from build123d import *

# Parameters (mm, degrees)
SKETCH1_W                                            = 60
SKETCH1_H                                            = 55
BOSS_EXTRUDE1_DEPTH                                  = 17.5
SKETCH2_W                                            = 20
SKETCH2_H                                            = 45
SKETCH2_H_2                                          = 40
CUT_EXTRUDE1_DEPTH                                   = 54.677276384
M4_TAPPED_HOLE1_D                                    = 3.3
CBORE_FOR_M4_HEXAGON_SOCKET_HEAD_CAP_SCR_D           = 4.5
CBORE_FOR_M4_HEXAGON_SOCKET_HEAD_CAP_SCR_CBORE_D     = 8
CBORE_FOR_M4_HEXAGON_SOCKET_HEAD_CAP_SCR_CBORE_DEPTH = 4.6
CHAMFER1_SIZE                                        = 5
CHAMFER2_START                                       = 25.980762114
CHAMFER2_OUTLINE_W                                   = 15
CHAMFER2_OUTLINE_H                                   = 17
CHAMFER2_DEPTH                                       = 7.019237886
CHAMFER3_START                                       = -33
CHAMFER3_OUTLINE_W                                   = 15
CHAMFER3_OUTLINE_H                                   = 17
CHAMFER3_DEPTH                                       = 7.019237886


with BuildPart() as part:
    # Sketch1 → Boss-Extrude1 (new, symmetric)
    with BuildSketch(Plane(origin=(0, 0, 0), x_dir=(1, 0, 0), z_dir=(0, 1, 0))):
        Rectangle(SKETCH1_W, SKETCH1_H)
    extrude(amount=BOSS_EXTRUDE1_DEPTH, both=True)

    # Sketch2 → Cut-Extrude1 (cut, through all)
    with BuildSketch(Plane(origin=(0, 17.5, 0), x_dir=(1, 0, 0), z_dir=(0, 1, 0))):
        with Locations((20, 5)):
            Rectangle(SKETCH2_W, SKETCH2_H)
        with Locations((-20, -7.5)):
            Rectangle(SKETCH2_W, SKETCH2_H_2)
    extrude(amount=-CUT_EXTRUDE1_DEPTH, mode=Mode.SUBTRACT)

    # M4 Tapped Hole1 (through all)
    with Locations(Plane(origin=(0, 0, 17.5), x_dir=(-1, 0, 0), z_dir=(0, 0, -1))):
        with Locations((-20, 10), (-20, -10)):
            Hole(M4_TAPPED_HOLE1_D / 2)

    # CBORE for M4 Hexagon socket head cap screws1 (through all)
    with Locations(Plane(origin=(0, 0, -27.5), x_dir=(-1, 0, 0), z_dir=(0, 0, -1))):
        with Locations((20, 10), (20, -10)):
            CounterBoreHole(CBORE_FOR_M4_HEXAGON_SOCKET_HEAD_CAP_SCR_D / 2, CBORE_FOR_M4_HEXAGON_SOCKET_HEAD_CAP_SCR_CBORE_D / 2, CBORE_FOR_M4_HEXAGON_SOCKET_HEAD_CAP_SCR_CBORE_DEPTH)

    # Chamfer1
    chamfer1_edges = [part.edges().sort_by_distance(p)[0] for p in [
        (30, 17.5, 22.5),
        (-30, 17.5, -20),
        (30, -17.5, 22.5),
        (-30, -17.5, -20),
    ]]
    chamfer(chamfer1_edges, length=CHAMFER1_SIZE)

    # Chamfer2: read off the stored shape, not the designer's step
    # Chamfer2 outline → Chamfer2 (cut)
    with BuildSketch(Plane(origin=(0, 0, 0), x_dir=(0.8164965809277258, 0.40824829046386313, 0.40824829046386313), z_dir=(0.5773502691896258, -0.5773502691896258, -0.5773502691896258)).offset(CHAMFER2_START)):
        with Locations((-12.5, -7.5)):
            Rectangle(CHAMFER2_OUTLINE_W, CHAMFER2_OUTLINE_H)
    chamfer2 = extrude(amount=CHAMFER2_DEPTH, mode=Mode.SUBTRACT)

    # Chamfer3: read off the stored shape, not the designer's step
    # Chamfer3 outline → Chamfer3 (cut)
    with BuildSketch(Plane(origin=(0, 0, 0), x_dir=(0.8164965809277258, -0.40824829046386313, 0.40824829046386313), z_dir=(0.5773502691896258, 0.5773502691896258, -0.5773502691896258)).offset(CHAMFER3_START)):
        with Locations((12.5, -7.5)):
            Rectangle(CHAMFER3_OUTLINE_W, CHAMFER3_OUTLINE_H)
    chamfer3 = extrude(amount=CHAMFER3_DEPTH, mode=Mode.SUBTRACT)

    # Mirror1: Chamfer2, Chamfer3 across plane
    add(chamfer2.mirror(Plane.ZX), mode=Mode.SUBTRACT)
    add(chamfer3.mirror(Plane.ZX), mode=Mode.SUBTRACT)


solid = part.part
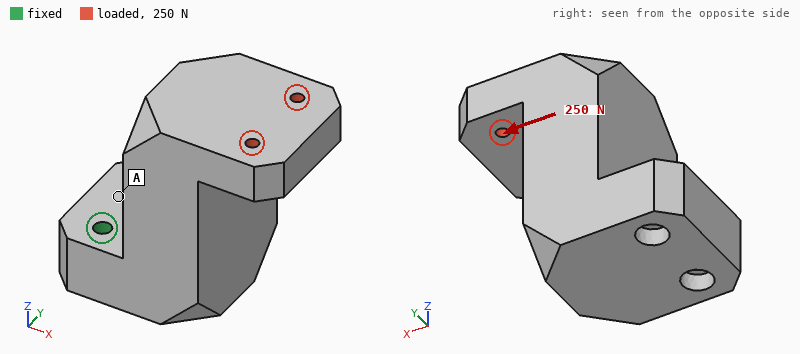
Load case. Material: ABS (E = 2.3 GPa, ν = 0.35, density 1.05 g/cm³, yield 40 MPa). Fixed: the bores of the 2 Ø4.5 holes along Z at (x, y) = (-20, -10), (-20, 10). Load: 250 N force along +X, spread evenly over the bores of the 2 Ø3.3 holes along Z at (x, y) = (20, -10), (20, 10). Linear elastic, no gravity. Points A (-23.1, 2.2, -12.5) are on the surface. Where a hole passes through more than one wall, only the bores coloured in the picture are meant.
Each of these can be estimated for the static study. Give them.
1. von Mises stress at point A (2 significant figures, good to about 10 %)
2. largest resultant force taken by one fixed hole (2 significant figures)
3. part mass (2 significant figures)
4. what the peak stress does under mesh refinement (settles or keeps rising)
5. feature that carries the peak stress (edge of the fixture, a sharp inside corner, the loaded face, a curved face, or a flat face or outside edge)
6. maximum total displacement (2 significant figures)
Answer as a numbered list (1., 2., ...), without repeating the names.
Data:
1. 2.5 MPa
2. 140 N
3. 56 g
4. keeps rising
5. edge of the fixture
6. 0.91 mm
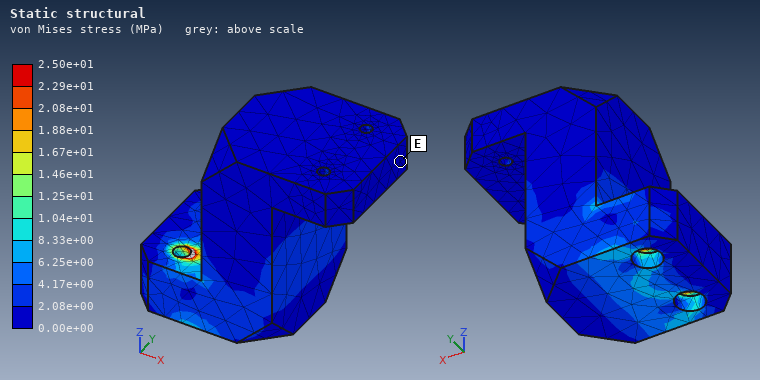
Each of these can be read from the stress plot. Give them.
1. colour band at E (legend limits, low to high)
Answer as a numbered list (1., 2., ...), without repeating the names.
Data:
1. 0.00e+00 to 2.08e+00 MPa
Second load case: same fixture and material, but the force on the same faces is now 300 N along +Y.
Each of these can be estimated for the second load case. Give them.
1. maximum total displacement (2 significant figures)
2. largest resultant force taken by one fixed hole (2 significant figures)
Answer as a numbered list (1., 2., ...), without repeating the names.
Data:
1. 0.52 mm
2. 720 N
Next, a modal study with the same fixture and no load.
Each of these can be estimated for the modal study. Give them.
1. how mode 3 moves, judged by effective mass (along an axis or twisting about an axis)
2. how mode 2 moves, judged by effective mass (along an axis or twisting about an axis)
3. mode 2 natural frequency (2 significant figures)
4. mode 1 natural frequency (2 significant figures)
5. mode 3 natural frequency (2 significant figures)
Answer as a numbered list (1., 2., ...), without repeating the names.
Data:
1. twisting about Z
2. along Y
3. 1000 Hz
4. 610 Hz
5. 2400 Hz
